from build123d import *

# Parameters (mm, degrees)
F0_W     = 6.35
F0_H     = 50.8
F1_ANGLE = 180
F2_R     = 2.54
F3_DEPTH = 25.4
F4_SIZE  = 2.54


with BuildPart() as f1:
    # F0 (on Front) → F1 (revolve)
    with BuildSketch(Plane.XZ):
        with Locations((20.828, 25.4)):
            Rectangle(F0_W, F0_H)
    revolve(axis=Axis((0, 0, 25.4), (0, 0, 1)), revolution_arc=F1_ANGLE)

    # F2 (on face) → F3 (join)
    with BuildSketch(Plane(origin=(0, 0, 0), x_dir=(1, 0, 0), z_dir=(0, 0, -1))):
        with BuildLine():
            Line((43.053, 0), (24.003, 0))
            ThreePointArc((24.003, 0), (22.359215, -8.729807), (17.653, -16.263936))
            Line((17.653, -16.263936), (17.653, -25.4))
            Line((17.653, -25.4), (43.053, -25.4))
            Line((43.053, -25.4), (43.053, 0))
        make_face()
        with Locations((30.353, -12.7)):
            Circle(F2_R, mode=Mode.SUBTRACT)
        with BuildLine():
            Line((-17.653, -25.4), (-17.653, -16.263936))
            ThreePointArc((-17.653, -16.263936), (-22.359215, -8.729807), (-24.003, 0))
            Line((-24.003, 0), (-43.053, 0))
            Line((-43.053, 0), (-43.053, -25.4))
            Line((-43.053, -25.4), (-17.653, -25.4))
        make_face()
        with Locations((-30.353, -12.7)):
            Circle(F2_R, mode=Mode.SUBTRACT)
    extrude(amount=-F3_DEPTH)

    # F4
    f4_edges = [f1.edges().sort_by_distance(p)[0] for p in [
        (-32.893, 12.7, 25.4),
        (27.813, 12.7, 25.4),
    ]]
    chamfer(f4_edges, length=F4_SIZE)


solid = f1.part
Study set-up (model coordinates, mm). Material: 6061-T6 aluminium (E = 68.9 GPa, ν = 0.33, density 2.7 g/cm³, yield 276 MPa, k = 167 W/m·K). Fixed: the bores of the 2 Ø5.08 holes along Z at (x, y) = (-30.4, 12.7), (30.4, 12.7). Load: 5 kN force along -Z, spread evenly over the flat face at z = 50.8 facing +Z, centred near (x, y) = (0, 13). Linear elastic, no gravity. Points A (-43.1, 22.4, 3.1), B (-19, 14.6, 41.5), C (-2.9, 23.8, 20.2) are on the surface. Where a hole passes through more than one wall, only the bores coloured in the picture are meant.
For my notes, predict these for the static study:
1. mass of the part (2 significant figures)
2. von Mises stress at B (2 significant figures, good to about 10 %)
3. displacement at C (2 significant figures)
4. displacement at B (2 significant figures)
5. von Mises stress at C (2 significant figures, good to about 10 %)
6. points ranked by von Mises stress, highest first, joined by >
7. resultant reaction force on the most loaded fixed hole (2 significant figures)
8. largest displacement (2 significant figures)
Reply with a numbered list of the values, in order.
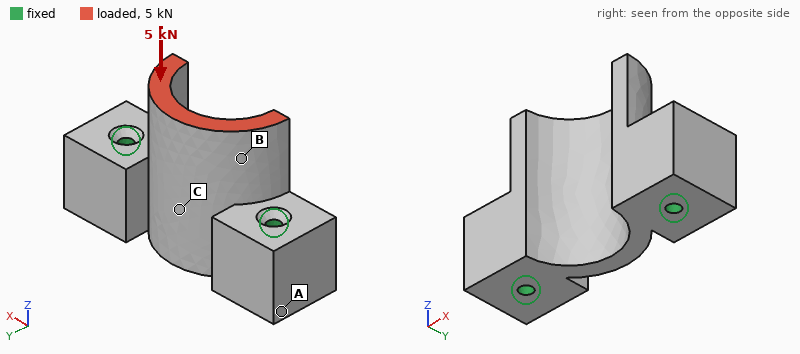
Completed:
1. 130 g
2. 13 MPa
3. 12 µm
4. 12 µm
5. 7.5 MPa
6. B > C > A
7. 2.5 kN
8. 24 µm
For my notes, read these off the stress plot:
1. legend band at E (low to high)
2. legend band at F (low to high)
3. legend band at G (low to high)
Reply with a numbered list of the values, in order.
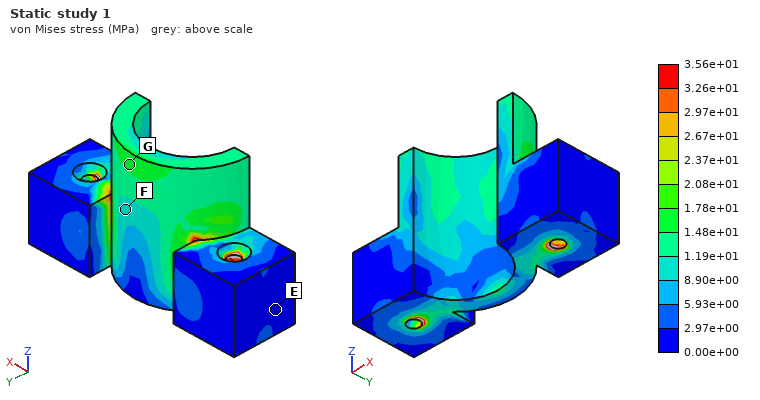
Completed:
1. 0.00e+00 to 2.97e+00 MPa
2. 8.90e+00 to 1.19e+01 MPa
3. 1.48e+01 to 1.78e+01 MPa
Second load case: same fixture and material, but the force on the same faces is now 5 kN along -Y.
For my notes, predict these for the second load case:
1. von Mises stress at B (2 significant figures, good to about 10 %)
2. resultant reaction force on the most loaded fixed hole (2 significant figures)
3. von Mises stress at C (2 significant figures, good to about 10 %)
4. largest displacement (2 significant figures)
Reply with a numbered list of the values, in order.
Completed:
1. 60 MPa
2. 2.8 kN
3. 45 MPa
4. 0.17 mm
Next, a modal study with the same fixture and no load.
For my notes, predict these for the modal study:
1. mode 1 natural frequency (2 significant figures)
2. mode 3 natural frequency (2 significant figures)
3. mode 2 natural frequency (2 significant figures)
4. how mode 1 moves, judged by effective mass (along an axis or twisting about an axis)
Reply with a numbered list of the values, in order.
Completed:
1. 7600 Hz
2. 12 kHz
3. 8600 Hz
4. along Y
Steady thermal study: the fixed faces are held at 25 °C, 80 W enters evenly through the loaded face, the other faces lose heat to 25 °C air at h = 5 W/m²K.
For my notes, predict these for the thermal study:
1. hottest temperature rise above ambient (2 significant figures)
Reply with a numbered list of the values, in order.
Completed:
1. 45 K
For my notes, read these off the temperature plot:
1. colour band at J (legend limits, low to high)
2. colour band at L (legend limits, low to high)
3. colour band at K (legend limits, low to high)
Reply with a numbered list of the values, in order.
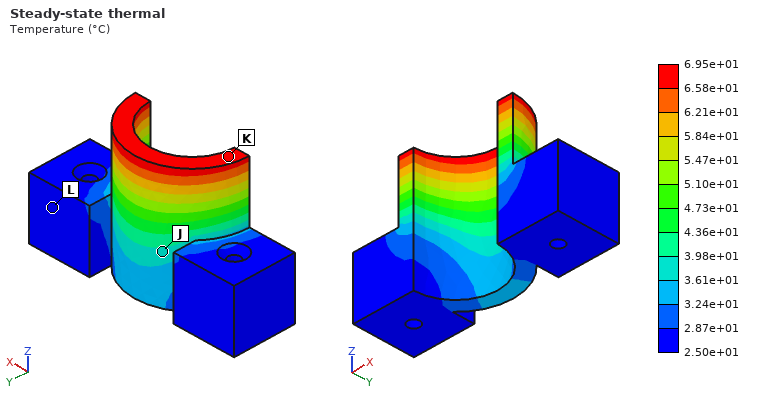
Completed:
1. 3.61e+01 to 3.98e+01 °C
2. 2.50e+01 to 2.87e+01 °C
3. 6.58e+01 to 6.95e+01 °C
